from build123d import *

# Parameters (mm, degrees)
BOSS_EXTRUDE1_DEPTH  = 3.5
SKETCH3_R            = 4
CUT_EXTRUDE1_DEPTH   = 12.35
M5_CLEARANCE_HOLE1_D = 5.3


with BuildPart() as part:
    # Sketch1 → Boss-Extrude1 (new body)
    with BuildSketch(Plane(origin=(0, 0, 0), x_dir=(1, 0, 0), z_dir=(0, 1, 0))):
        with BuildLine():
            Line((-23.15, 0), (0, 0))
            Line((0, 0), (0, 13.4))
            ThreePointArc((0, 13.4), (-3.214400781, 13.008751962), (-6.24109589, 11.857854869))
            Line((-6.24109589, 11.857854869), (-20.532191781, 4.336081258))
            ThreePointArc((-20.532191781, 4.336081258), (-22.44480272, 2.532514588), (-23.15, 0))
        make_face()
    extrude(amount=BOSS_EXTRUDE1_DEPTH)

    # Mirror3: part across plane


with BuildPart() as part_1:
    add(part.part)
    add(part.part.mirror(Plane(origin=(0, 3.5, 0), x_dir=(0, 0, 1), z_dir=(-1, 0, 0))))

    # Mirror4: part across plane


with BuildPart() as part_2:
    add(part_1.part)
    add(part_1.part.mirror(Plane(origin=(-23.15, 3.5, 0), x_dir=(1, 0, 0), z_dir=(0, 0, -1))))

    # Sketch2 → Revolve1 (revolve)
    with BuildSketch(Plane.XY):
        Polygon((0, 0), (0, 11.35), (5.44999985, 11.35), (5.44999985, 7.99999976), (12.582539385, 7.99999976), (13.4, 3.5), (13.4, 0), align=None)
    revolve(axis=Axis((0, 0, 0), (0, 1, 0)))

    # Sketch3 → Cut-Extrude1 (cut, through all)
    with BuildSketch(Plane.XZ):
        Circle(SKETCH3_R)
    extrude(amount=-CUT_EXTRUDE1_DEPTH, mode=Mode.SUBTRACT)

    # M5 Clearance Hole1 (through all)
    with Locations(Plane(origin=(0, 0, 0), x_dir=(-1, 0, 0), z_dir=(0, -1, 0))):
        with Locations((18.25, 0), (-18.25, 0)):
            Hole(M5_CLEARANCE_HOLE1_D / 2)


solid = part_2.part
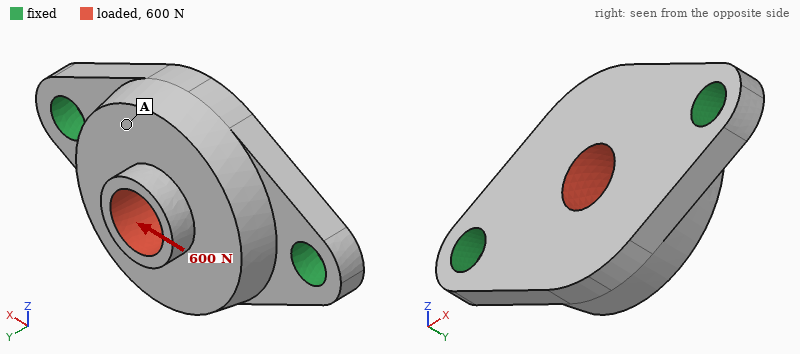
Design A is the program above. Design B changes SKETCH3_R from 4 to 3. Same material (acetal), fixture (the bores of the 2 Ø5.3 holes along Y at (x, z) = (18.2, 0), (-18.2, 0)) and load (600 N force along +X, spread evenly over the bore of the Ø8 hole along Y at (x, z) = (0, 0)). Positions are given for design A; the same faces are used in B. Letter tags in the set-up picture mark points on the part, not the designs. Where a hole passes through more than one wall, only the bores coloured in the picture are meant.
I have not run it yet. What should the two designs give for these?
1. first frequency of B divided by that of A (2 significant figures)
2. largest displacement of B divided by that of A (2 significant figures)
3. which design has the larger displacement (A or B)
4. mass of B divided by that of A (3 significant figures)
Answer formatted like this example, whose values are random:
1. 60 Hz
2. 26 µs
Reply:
1. 0.99
2. 0.82
3. A
4. 1.05
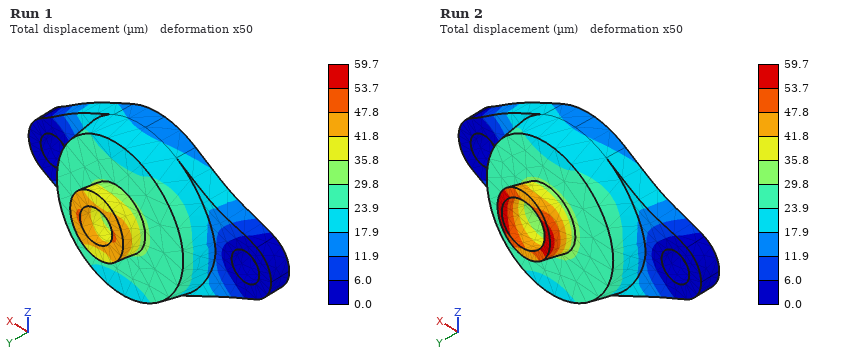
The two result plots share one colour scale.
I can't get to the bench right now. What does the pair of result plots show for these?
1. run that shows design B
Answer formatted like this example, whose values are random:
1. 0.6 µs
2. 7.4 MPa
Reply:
1. Run 1
